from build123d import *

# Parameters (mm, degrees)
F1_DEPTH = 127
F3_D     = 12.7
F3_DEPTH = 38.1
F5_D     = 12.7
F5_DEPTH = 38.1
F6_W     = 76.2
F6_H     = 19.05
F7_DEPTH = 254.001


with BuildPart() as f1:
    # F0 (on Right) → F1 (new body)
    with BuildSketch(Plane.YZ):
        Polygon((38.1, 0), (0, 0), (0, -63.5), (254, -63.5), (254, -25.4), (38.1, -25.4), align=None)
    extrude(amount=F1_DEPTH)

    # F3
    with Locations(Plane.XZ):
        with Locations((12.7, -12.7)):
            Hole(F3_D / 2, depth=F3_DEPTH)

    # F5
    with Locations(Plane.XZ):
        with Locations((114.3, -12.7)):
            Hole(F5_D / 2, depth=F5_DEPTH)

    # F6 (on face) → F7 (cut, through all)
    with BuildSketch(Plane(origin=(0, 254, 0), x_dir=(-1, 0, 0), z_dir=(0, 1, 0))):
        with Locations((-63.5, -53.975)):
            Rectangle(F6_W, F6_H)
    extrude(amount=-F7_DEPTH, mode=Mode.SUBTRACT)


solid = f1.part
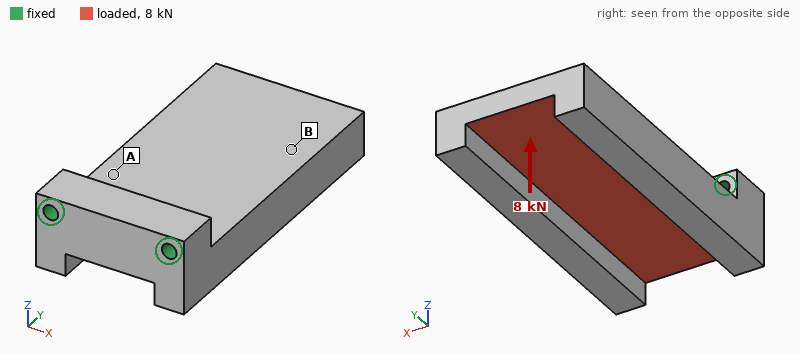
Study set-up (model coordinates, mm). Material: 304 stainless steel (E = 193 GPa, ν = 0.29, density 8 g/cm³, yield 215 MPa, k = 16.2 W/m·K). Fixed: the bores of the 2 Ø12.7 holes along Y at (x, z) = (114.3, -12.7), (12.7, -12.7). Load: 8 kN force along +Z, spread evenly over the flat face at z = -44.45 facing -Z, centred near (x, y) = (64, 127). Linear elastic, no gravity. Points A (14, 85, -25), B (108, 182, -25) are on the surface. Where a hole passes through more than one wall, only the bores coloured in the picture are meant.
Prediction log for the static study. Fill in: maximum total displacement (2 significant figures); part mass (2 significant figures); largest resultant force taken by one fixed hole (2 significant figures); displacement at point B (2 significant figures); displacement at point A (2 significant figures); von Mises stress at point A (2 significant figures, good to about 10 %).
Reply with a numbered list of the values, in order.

1. 0.25 mm
2. 7.8 kg
3. 4.9 kN
4. 0.15 mm
5. 0.041 mm
6. 20 MPa
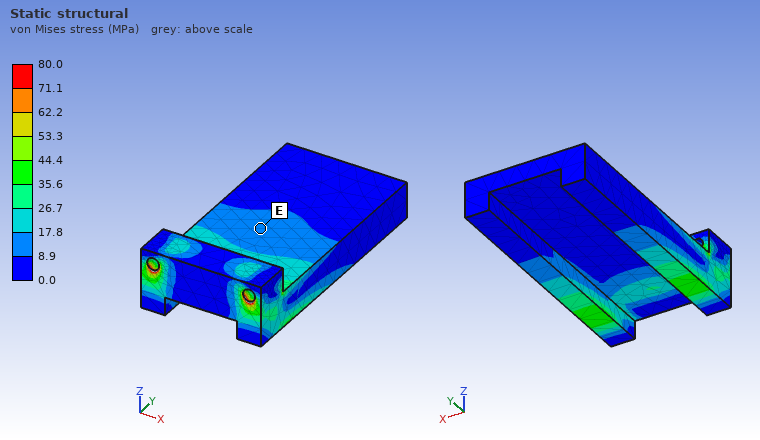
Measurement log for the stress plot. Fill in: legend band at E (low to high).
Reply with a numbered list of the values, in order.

1. 8.9 to 17.8 MPa
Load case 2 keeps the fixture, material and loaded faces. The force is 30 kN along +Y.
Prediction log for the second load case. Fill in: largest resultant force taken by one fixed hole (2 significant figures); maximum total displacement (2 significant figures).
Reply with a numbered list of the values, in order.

1. 15 kN
2. 100 µm
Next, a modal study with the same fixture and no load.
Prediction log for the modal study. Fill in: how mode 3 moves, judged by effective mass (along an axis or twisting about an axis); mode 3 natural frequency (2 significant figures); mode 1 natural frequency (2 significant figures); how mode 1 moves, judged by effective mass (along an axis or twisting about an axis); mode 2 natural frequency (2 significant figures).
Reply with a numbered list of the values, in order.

1. along X
2. 1200 Hz
3. 430 Hz
4. along Z
5. 1100 Hz
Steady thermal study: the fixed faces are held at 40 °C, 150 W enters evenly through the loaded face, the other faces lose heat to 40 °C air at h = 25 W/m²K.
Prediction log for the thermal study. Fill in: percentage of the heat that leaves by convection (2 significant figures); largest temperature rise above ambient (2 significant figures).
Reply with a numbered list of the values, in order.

1. 67 %
2. 84 K
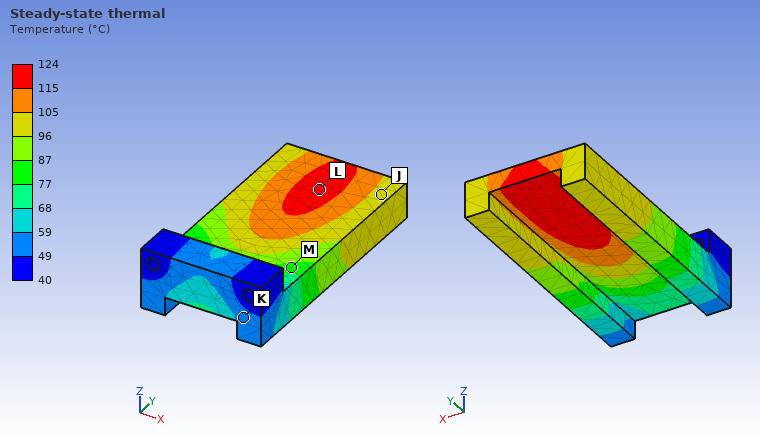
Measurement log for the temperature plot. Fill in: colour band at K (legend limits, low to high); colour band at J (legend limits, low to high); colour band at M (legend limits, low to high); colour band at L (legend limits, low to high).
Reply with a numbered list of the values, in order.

1. 49 to 59 °C
2. 96 to 105 °C
3. 77 to 87 °C
4. 115 to 124 °C
